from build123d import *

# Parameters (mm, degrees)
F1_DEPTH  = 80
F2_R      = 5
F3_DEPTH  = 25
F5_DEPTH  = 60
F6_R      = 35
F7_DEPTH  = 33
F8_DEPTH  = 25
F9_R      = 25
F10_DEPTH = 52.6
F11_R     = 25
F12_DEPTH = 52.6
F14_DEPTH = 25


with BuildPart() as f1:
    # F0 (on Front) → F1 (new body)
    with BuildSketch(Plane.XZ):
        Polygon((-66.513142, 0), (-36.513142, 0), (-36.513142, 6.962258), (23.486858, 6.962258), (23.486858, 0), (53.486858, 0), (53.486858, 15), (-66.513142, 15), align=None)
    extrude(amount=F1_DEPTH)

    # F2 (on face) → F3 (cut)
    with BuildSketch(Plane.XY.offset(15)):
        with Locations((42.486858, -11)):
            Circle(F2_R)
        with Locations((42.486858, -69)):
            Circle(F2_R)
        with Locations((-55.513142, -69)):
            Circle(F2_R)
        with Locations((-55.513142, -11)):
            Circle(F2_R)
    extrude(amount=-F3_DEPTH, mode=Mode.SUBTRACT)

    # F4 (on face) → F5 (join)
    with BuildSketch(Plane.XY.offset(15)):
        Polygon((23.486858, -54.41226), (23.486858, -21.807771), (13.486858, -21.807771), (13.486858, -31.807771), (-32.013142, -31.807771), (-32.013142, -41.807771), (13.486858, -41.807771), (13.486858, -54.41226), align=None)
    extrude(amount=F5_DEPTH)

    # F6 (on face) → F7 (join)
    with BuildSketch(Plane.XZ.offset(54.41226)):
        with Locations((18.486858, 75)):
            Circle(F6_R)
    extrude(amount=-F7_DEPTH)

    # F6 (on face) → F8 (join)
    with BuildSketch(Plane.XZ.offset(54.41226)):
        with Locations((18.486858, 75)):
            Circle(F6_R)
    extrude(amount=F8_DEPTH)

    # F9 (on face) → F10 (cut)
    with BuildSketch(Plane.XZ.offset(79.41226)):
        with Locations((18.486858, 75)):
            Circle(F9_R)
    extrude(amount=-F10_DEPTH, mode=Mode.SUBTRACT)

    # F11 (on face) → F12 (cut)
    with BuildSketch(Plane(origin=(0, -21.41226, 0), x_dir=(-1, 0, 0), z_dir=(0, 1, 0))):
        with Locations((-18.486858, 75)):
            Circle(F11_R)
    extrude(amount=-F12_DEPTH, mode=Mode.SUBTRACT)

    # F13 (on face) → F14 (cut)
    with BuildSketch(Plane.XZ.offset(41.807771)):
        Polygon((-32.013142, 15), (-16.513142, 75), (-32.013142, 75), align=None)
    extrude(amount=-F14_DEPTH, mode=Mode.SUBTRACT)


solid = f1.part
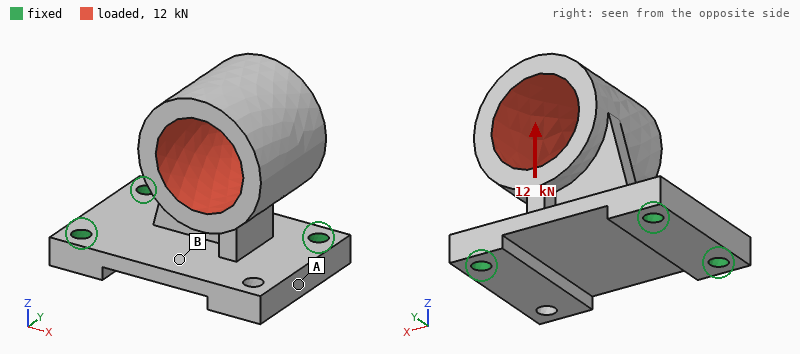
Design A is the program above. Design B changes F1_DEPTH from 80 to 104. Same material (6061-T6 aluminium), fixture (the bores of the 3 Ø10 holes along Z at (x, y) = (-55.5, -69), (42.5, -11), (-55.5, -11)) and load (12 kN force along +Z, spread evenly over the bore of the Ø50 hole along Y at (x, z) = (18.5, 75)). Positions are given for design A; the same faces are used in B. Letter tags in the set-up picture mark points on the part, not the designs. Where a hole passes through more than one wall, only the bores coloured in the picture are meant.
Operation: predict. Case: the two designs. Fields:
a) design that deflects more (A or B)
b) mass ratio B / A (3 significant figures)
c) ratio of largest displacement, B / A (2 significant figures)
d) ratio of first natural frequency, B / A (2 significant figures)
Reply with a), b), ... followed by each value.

a) A
b) 1.14
c) 0.87
d) 1.0
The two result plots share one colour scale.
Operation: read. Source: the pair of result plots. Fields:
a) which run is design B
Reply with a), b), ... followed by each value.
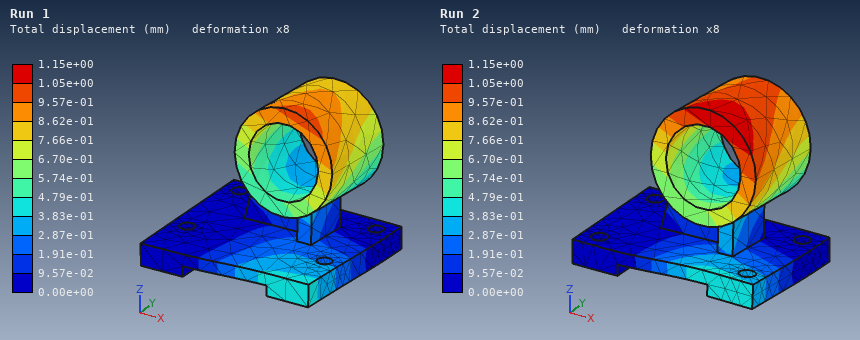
a) Run 1
